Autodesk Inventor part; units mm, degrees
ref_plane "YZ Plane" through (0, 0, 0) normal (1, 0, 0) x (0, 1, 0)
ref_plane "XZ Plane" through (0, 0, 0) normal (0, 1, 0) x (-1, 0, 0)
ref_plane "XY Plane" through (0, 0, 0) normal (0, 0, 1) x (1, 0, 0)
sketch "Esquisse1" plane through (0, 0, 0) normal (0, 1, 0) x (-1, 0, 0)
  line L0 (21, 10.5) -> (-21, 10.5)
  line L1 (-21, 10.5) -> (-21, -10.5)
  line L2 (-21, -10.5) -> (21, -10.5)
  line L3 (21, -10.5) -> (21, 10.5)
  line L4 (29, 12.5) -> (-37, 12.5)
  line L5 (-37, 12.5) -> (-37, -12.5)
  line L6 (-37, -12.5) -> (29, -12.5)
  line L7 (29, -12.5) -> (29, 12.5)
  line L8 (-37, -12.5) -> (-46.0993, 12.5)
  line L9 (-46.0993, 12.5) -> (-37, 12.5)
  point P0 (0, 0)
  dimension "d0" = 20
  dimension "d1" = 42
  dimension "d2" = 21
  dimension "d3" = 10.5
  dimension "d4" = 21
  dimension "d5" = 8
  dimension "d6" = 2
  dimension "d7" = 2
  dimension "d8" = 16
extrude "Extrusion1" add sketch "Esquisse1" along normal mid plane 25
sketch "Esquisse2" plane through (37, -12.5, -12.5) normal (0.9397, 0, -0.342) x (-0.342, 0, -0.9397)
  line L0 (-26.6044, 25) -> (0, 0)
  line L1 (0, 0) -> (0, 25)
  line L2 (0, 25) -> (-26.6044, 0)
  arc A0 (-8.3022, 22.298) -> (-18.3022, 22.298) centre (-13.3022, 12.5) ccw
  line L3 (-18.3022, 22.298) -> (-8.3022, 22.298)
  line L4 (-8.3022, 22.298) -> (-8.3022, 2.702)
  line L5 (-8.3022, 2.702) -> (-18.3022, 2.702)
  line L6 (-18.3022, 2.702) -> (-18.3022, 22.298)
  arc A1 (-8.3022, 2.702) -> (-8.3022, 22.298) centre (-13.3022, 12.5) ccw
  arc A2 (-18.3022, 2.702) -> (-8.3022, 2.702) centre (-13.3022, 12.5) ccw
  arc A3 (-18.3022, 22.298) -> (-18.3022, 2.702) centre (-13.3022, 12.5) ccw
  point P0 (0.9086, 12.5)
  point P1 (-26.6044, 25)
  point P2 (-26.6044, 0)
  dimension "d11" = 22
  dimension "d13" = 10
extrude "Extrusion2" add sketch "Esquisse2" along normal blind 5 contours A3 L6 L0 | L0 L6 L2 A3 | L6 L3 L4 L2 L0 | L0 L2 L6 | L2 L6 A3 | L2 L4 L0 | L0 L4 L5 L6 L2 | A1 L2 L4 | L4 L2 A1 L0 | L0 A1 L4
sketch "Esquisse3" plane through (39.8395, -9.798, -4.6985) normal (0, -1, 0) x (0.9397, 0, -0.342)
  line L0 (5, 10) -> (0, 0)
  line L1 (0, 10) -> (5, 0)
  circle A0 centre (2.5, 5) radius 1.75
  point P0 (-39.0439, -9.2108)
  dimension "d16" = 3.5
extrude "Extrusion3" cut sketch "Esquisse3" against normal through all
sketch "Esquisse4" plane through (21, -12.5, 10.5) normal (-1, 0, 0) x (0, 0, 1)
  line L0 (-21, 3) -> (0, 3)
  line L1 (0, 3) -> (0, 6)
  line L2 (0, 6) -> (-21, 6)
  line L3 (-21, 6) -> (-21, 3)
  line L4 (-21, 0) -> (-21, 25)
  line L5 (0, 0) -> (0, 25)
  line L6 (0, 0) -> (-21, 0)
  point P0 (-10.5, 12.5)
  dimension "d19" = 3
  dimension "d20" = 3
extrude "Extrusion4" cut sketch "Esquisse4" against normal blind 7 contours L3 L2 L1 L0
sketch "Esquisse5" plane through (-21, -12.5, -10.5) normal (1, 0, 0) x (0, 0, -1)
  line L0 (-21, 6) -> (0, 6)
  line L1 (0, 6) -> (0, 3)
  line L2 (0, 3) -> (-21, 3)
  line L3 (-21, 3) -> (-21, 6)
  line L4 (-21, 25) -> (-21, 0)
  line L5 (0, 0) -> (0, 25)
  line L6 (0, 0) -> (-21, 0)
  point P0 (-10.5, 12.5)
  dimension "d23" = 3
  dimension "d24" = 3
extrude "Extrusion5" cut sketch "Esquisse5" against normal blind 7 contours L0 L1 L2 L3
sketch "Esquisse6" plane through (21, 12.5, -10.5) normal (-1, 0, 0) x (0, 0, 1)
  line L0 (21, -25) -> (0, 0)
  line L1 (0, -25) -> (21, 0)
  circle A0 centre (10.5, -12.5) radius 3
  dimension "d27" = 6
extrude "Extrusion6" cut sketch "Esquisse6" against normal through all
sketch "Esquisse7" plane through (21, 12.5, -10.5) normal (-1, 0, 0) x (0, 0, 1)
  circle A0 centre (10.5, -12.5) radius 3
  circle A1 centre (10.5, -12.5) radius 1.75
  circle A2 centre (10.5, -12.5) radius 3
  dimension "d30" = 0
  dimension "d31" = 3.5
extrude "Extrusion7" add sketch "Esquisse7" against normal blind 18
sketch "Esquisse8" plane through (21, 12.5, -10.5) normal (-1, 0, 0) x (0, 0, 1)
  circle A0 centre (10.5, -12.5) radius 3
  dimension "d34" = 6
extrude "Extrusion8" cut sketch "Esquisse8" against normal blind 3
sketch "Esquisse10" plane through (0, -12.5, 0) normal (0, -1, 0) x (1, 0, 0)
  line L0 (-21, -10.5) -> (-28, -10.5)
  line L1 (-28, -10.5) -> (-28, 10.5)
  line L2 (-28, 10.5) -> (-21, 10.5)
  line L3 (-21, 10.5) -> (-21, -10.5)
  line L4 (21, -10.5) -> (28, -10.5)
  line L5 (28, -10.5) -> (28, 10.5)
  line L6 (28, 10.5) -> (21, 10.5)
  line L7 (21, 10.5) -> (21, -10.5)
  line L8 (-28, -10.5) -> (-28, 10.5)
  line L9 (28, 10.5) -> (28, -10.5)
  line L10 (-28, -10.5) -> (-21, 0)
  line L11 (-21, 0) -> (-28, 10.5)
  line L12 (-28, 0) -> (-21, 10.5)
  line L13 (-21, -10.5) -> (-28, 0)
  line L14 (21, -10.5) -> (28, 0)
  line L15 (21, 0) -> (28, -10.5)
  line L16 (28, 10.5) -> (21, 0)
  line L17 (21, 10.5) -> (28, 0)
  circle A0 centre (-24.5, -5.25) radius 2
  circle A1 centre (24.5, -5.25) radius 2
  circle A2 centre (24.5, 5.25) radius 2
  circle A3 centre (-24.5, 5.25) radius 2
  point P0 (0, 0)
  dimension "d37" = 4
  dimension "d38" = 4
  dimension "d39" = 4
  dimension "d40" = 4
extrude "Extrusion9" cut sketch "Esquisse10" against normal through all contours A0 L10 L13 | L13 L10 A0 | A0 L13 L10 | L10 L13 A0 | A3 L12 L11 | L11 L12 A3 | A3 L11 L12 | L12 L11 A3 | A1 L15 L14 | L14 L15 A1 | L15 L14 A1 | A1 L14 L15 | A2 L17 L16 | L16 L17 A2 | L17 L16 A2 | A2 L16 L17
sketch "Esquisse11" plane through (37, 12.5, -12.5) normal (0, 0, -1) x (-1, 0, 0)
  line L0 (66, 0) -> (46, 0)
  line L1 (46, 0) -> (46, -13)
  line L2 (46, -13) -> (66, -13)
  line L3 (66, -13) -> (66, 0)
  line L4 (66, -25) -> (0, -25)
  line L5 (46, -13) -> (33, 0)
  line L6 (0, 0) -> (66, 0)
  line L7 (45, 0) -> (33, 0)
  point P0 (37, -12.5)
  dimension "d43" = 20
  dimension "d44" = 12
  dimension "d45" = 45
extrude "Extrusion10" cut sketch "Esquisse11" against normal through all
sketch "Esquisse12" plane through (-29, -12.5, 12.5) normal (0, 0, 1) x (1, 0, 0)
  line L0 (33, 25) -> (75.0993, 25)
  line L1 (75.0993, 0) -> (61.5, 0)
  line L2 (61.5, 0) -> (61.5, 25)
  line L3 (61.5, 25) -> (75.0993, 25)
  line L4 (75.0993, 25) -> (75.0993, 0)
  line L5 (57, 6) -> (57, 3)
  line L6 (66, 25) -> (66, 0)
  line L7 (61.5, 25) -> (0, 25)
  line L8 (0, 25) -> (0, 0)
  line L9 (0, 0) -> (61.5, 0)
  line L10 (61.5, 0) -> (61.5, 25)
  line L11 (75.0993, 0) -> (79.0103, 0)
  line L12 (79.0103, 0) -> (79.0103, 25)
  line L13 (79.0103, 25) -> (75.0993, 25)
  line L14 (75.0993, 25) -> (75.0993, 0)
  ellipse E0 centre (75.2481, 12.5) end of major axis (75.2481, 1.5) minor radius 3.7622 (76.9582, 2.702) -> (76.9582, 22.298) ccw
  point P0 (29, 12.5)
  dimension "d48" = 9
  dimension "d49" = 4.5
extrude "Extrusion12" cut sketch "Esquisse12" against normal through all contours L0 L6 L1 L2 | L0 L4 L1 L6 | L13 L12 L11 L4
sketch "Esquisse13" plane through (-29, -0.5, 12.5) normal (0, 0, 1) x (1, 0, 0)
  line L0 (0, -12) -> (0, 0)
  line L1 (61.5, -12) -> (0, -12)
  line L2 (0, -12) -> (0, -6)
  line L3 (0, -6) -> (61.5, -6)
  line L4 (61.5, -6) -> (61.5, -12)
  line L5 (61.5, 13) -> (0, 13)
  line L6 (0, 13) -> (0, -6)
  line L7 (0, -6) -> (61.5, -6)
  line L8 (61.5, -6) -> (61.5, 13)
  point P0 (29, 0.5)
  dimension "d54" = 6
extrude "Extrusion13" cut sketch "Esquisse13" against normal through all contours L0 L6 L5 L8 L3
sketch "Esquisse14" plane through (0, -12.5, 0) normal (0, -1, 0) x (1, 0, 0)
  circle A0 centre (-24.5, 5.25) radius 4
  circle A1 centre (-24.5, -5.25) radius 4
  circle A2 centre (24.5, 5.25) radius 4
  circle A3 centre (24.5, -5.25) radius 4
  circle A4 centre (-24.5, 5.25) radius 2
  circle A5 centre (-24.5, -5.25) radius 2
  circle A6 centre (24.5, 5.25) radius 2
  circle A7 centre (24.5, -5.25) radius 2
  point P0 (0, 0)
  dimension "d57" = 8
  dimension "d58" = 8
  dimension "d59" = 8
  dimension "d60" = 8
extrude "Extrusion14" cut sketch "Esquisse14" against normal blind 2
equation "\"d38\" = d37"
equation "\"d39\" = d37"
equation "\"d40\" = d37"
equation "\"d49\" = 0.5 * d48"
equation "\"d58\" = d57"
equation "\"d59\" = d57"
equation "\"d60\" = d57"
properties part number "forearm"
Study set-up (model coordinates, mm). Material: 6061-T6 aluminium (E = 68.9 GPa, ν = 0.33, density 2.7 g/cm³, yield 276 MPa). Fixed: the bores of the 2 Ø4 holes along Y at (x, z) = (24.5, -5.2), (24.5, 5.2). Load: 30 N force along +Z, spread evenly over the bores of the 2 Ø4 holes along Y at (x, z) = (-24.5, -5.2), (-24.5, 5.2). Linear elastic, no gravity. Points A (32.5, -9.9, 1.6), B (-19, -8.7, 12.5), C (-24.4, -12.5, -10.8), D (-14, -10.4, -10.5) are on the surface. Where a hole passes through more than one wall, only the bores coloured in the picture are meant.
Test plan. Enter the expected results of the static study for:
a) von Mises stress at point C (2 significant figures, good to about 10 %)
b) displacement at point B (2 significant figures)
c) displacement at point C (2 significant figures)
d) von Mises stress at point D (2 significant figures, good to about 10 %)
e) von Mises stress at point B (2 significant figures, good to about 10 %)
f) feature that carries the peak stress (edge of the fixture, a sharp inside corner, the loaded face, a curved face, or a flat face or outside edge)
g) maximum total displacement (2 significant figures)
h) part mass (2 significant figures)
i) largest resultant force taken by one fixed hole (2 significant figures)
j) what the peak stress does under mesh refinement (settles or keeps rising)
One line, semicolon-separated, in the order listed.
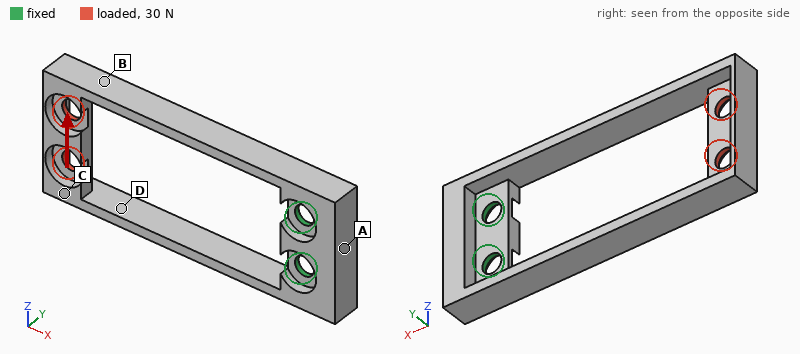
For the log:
12 MPa; 0.44 mm; 0.45 mm; 55 MPa; 64 MPa; a sharp inside corner; 0.46 mm; 7.0 g; 92 N; keeps rising
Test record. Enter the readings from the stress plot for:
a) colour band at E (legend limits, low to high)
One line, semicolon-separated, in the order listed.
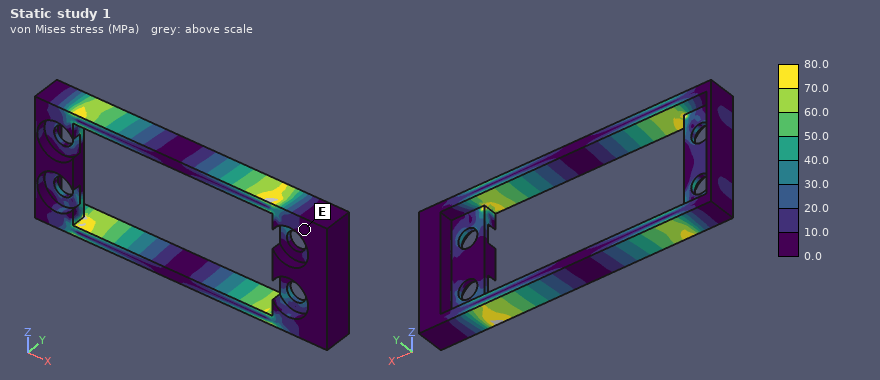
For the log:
0.0 to 10.0 MPa
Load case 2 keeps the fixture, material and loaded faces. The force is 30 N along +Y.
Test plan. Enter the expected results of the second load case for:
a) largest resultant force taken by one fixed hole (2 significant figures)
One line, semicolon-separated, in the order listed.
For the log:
17 N
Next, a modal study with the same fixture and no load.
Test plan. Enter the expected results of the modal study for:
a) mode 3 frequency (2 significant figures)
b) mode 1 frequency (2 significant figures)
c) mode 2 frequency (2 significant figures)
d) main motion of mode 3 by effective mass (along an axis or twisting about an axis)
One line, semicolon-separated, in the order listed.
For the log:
1900 Hz; 830 Hz; 830 Hz; twisting about X
